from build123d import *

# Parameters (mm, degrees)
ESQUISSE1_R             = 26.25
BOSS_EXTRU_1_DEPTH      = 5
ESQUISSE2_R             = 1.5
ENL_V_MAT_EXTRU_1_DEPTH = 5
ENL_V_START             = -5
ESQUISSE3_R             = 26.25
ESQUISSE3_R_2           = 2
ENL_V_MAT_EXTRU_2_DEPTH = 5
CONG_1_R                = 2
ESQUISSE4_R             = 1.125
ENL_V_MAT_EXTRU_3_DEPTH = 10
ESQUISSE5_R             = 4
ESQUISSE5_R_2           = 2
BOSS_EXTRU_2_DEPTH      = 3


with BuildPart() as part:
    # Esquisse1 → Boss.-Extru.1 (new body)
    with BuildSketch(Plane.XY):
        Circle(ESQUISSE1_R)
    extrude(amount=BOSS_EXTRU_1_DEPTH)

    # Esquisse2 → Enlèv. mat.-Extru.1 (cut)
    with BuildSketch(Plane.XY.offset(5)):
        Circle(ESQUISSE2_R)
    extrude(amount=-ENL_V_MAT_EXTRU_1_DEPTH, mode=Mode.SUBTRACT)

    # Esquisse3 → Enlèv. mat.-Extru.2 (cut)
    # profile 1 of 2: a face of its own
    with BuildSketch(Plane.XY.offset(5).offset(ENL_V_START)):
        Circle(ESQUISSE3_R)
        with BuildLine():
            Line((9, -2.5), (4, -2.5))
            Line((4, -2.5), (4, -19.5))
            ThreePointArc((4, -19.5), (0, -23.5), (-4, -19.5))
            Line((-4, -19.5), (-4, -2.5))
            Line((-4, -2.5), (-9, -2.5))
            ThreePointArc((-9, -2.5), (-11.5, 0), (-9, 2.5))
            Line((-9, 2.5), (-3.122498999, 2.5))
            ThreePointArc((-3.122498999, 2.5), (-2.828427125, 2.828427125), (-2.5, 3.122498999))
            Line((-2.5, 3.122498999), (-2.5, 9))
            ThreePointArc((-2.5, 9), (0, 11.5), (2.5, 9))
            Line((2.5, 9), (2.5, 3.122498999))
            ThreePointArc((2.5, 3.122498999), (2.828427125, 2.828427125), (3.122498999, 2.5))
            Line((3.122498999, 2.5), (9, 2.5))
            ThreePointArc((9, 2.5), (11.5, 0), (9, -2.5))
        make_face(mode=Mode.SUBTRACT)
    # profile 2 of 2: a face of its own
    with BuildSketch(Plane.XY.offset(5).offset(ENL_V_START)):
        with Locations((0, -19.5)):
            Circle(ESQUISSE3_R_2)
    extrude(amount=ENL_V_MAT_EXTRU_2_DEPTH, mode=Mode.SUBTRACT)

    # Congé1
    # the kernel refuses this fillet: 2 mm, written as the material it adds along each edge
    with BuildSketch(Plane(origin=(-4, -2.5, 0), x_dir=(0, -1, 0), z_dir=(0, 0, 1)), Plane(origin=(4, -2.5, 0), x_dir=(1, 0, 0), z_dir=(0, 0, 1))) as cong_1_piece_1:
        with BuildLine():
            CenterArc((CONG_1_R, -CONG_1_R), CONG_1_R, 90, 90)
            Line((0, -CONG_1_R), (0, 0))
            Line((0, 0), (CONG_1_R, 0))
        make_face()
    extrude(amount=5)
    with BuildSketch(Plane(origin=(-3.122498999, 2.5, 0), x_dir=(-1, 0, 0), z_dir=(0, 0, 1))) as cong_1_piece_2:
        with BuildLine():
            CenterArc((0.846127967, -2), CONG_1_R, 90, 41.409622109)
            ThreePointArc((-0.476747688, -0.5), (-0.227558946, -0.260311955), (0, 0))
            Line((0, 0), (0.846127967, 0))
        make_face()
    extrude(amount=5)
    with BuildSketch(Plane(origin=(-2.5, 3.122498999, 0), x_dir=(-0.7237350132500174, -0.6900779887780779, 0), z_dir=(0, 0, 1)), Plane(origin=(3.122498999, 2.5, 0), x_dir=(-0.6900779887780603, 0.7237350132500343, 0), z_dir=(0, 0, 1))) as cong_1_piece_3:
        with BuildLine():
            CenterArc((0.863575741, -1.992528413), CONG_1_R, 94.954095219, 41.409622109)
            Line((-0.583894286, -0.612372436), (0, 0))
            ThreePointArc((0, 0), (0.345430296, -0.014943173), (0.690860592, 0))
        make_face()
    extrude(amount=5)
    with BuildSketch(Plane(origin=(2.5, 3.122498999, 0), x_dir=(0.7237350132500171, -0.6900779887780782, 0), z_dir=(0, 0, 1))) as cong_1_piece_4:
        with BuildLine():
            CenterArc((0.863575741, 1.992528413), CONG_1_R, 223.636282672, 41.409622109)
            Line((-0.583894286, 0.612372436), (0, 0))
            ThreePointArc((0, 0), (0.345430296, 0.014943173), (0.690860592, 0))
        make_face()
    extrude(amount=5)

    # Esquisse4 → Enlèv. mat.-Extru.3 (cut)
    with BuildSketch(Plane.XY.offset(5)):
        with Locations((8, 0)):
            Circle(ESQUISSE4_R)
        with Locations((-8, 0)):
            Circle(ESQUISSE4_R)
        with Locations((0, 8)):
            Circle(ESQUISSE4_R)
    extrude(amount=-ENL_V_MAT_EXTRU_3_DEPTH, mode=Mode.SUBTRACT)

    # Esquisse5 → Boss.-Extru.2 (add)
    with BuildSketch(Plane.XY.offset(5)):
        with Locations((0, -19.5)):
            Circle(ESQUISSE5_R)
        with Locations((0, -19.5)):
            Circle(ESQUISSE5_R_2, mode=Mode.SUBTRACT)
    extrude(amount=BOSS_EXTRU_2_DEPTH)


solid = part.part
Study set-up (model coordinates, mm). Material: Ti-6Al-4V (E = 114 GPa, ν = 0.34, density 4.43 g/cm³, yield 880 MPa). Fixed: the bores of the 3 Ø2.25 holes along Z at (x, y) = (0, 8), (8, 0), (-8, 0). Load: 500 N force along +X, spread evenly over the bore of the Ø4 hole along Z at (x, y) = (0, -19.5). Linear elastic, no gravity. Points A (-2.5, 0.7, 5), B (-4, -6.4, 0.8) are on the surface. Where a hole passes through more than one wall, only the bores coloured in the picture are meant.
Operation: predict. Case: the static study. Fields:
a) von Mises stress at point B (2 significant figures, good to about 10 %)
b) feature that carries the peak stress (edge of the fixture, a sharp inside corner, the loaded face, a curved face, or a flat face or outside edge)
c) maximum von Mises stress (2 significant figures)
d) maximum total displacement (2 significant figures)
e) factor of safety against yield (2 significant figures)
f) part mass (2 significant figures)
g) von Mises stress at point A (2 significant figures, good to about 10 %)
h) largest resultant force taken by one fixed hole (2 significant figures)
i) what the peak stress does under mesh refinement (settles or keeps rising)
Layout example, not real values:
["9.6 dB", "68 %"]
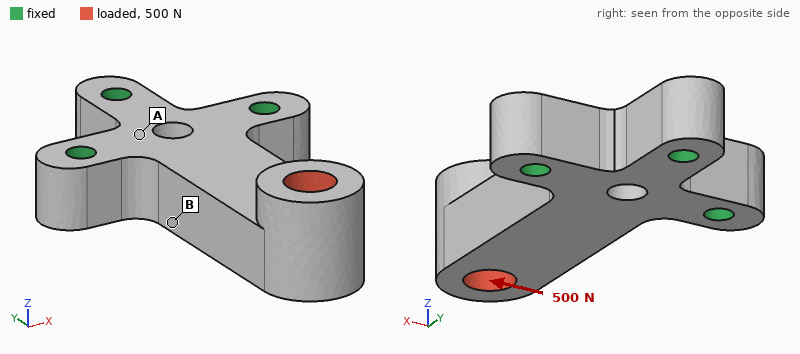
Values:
["120 MPa", "a curved face", "240 MPa", "76 µm", "3.7", "6.8 g", "40 MPa", "710 N", "settles"]
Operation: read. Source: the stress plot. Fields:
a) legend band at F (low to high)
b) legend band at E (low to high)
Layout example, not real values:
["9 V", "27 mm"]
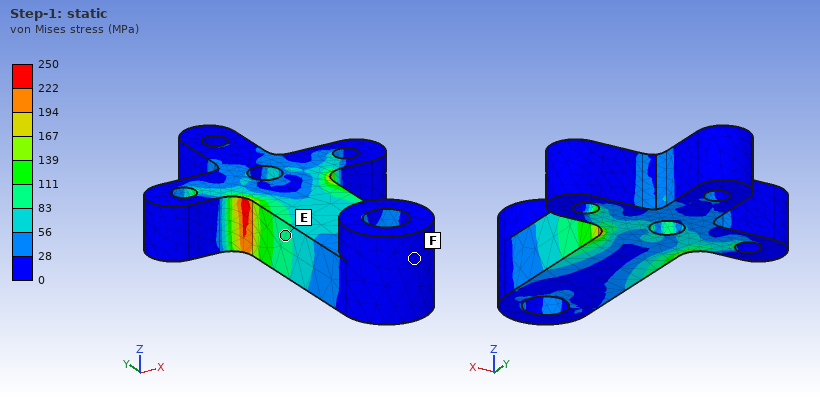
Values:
["0 to 28 MPa", "83 to 111 MPa"]
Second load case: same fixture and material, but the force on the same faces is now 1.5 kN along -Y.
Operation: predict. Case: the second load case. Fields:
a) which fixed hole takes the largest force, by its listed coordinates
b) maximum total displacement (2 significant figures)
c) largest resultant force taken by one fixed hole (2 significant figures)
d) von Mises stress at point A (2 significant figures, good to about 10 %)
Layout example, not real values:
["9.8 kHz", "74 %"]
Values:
["(0, 8)", "84 µm", "690 N", "62 MPa"]
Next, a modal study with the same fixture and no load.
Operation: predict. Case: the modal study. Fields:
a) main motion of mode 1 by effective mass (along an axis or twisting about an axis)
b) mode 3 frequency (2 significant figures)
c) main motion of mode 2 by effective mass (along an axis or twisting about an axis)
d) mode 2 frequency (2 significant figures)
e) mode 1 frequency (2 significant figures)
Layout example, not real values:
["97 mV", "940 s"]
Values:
["along Z", "25 kHz", "along X", "11 kHz", "6000 Hz"]
